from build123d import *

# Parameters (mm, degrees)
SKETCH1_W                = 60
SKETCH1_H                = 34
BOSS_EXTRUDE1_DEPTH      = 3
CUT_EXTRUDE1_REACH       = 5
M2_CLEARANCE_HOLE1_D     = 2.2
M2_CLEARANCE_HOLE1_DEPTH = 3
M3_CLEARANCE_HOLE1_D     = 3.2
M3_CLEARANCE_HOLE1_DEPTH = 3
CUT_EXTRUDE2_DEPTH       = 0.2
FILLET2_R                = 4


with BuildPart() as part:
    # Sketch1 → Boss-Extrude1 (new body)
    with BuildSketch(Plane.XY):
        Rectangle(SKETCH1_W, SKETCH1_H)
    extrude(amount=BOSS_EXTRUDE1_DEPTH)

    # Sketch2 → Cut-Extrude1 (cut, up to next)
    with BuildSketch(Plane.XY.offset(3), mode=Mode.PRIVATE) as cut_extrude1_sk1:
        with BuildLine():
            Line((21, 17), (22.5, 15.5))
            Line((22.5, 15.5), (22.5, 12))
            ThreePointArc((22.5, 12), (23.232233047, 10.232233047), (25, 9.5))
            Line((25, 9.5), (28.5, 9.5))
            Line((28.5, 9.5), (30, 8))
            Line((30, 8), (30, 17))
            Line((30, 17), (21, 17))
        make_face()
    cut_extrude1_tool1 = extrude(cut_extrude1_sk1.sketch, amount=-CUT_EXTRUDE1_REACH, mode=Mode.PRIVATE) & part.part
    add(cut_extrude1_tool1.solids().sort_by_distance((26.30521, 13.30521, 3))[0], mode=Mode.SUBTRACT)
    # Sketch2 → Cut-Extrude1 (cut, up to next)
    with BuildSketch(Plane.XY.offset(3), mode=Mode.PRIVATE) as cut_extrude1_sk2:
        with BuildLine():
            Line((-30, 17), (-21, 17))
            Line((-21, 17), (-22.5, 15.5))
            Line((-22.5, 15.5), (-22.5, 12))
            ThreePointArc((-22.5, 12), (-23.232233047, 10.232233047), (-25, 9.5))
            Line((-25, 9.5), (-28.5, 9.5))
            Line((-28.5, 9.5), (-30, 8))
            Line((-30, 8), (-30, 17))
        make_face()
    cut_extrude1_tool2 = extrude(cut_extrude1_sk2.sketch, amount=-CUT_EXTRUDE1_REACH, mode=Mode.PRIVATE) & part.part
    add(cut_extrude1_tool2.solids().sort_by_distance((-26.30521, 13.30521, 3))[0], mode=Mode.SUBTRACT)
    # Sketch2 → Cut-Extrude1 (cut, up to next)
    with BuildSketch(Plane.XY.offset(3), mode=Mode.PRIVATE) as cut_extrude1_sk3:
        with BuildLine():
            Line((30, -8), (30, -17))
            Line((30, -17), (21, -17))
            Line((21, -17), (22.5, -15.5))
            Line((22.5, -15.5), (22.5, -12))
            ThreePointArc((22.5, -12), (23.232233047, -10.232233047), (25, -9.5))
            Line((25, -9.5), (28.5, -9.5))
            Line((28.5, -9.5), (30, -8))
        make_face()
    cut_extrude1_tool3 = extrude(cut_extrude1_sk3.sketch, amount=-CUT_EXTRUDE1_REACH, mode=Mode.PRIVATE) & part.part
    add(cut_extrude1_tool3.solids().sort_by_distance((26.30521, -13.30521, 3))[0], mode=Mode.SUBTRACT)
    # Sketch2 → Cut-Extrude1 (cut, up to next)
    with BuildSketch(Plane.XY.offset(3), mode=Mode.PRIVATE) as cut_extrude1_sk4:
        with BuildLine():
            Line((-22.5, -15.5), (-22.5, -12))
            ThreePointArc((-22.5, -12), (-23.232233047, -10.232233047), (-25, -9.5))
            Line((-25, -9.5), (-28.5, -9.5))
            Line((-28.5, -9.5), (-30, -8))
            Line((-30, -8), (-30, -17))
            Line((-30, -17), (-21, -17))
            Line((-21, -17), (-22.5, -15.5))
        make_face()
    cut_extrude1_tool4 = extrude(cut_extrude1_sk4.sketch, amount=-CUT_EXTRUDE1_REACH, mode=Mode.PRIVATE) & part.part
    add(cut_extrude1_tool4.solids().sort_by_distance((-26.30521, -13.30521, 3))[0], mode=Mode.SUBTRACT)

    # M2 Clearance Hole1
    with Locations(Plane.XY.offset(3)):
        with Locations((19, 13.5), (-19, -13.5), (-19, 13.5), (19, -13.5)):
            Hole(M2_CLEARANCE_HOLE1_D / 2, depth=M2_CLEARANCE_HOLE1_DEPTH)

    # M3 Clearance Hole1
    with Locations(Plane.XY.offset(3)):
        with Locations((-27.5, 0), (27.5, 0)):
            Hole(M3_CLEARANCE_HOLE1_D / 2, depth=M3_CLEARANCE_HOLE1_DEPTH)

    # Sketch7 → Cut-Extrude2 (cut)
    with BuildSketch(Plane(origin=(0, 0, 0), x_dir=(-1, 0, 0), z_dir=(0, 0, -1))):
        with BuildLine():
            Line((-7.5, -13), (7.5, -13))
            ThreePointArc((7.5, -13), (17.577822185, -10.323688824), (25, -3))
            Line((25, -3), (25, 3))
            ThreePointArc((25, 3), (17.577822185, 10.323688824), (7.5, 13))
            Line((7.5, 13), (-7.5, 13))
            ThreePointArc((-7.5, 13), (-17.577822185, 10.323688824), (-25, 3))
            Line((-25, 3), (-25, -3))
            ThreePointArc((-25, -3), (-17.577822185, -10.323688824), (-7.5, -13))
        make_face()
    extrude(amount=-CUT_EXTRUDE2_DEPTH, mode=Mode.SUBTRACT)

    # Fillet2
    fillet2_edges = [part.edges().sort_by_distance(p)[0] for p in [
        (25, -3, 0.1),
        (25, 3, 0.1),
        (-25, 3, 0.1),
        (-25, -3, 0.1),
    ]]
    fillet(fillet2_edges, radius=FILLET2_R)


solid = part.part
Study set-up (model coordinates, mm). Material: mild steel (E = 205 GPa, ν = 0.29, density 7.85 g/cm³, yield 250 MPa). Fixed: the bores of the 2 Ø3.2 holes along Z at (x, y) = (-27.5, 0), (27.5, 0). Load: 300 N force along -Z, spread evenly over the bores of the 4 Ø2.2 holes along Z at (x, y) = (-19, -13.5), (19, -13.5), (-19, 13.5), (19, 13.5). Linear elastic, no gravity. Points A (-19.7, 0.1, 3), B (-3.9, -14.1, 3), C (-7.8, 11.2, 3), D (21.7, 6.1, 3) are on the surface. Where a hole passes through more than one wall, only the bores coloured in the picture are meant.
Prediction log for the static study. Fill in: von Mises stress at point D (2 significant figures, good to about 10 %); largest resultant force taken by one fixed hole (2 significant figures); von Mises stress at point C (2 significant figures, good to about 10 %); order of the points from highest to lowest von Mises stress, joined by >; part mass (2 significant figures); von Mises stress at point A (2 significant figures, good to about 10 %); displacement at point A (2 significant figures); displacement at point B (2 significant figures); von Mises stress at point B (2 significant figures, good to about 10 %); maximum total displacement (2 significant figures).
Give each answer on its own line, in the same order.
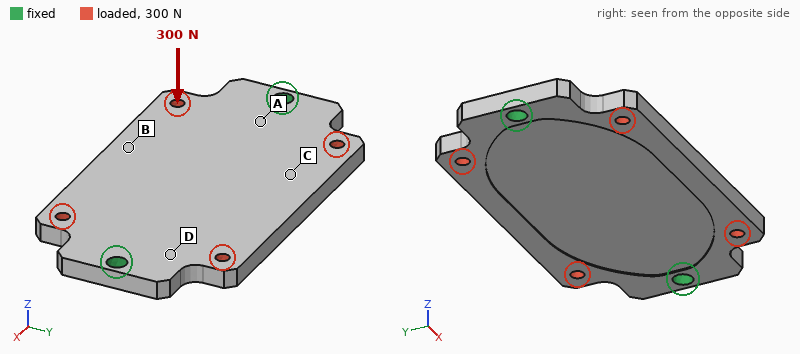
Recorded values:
18 MPa
150 N
9.9 MPa
A > D > C > B
40 g
26 MPa
3.2 µm
13 µm
5.5 MPa
14 µm
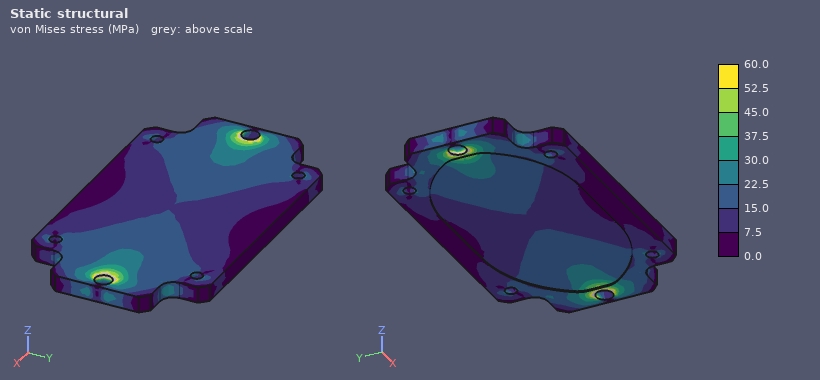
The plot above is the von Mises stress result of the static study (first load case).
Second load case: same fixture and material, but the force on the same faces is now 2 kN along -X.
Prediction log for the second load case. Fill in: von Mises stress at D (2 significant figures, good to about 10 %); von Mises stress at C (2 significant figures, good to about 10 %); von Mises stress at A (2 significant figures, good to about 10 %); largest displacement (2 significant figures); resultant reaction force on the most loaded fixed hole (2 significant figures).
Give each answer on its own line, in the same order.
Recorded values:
17 MPa
8.2 MPa
21 MPa
3.2 µm
1.0 kN
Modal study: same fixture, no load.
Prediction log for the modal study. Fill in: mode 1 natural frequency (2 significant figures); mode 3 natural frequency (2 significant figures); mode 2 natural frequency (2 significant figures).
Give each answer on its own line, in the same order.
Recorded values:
3800 Hz
9400 Hz
3800 Hz
